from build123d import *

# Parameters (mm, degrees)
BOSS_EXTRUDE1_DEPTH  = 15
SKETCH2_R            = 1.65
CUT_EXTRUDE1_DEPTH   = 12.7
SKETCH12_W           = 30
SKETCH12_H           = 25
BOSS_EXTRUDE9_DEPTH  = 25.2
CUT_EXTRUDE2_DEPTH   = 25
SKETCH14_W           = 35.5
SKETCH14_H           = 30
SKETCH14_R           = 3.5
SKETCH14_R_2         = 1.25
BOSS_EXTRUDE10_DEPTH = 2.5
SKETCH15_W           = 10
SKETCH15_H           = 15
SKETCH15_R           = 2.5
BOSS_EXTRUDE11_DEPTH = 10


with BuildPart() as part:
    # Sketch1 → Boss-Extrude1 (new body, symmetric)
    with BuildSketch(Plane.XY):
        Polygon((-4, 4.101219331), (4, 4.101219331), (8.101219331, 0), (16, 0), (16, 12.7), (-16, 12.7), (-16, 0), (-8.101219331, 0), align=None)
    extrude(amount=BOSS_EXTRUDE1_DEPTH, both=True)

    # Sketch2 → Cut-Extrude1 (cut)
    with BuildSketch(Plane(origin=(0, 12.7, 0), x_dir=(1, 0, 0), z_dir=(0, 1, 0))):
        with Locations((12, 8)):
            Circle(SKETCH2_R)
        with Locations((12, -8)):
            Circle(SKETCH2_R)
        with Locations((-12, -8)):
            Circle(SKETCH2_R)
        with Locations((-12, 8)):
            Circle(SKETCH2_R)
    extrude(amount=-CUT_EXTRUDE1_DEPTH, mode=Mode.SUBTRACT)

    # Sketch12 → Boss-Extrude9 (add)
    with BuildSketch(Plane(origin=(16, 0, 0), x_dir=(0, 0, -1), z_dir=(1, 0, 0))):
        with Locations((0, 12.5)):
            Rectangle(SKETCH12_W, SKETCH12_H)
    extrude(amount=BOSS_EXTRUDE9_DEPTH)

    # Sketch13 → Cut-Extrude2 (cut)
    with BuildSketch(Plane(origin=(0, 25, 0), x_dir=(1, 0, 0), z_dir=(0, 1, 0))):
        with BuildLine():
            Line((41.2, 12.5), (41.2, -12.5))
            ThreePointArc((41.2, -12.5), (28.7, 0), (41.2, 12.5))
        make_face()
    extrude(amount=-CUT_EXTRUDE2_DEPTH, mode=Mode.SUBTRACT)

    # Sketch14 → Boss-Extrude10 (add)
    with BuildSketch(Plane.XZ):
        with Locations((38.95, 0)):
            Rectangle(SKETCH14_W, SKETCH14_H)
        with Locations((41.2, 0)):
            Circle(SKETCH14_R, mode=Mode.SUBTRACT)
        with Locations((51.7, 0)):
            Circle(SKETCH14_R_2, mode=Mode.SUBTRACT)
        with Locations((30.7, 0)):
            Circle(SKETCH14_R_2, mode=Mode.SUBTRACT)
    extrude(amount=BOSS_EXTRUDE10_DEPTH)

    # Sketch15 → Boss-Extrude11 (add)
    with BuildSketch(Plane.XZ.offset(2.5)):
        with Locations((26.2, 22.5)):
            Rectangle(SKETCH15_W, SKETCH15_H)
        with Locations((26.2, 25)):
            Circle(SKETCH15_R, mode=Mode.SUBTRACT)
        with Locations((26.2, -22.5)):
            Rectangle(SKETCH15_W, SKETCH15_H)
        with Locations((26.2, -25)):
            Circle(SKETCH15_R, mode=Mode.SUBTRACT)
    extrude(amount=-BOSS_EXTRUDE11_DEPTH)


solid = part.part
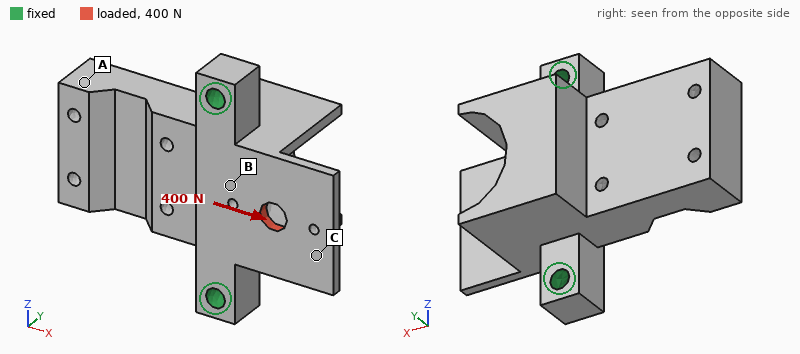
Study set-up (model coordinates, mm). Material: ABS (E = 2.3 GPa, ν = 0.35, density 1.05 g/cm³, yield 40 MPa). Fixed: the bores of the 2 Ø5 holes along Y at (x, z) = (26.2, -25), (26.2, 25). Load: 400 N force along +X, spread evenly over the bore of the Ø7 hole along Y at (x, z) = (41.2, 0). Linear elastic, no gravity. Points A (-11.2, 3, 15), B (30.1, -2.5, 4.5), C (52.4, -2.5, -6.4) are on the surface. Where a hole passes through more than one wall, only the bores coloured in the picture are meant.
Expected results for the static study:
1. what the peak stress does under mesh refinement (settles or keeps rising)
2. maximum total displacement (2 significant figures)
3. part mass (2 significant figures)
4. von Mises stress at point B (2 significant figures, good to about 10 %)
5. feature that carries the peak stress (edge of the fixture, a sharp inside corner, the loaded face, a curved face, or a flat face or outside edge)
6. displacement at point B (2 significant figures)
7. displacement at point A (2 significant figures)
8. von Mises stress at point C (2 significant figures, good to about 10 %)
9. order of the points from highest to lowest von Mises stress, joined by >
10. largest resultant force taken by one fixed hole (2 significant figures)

keeps rising
0.30 mm
30 g
4.3 MPa
edge of the fixture
0.11 mm
0.23 mm
2.4 MPa
B > C > A
200 N
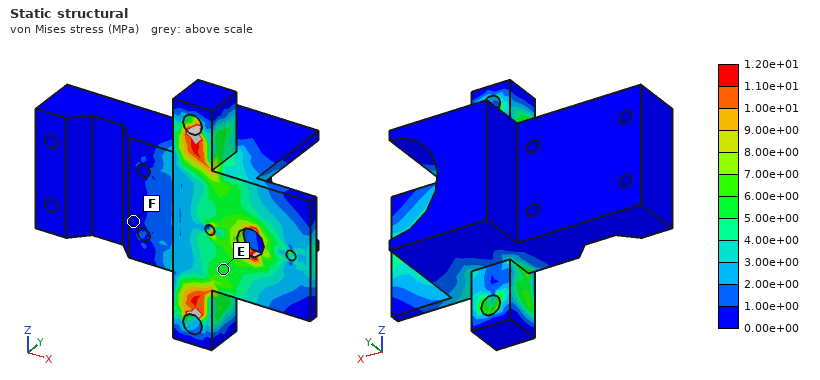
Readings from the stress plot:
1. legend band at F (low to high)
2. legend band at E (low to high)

0.00e+00 to 1.00e+00 MPa
5.00e+00 to 6.00e+00 MPa
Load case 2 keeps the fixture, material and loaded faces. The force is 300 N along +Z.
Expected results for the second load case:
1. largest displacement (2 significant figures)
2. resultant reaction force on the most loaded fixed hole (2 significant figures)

0.14 mm
190 N
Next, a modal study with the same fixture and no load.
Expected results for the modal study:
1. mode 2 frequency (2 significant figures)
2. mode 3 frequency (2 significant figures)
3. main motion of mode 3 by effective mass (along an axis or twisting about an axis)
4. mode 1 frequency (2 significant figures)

1400 Hz
2200 Hz
along Z
660 Hz
